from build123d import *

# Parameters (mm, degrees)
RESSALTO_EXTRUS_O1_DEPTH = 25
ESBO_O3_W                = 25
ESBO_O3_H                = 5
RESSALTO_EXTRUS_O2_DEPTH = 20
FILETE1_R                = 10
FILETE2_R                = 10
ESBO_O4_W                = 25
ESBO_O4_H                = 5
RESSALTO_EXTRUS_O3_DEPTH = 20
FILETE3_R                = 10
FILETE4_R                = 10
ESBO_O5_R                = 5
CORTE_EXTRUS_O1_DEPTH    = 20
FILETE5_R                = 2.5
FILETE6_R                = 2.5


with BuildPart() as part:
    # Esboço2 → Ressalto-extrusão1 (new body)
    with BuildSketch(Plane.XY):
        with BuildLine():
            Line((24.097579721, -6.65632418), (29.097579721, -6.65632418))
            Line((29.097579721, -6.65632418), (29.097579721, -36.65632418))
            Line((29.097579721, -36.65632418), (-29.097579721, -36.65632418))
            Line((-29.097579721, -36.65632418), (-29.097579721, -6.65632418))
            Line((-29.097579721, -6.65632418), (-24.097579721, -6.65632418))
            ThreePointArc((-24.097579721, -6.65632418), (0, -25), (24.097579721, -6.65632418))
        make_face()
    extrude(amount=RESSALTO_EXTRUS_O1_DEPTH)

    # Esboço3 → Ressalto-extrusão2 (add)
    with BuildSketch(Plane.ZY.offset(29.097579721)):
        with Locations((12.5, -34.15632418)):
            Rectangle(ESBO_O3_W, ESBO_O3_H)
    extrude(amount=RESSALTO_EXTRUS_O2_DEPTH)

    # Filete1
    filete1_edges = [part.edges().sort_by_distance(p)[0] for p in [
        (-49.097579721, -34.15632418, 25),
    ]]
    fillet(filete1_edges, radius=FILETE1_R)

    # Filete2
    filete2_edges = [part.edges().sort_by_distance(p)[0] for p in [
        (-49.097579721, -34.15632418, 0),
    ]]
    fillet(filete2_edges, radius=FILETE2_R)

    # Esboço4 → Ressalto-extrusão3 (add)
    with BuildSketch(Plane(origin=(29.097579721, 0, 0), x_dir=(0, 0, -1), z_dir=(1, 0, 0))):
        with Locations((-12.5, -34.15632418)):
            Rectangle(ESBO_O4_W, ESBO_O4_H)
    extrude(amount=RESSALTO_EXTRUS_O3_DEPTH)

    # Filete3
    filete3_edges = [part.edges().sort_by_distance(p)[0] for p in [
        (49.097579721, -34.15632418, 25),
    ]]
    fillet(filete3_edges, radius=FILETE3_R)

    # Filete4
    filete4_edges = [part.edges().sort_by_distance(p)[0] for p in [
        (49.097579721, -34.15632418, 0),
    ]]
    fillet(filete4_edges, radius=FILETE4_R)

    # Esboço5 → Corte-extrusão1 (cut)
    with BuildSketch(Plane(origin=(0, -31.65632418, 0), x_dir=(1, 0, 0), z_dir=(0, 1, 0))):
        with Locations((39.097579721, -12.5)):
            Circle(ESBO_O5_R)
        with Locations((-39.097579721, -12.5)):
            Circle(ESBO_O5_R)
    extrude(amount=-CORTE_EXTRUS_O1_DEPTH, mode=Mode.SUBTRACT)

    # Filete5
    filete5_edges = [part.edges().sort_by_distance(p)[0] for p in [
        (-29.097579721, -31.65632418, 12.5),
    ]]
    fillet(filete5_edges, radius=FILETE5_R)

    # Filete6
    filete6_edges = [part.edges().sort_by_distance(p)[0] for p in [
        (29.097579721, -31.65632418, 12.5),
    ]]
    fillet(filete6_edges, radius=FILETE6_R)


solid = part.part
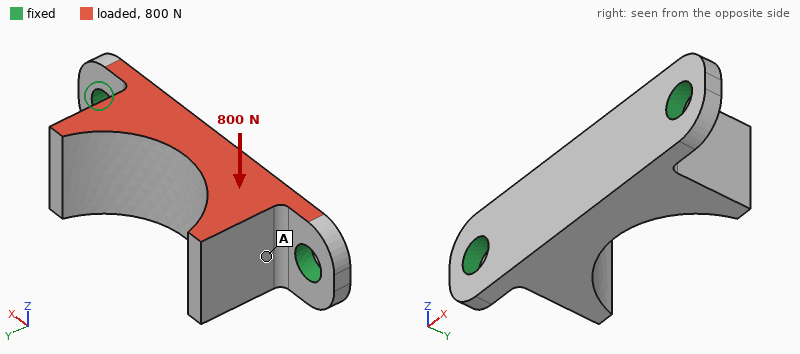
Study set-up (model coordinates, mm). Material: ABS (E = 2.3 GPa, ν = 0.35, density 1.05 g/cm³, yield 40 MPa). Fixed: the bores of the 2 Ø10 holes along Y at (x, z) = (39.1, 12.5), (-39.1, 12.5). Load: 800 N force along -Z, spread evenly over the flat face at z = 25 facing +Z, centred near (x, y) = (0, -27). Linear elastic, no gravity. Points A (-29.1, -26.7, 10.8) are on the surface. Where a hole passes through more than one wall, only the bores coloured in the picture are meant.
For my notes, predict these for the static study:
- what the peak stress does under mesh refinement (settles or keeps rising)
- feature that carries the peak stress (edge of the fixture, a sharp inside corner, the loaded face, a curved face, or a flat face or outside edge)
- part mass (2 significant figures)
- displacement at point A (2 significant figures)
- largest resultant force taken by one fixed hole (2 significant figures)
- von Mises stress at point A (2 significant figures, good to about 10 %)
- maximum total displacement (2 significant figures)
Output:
keeps rising
edge of the fixture
33 g
0.17 mm
400 N
4.4 MPa
0.55 mm
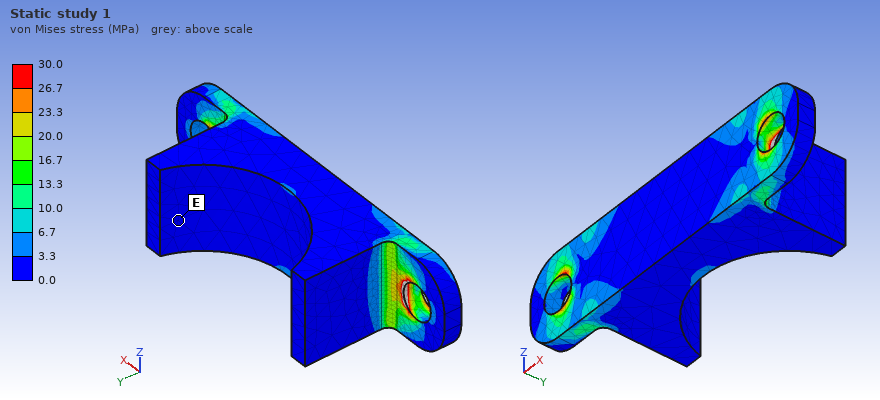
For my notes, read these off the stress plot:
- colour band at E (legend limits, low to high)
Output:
0.0 to 3.3 MPa
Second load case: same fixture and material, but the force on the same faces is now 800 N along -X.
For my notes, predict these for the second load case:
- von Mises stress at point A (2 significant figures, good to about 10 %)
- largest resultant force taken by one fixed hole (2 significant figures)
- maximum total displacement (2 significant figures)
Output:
1.4 MPa
430 N
94 µm
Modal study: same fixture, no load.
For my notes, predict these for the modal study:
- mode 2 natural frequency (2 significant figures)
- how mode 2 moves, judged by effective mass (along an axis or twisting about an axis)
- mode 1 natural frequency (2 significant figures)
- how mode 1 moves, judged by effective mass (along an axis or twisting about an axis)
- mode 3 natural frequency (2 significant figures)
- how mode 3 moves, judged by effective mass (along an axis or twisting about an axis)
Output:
1900 Hz
along Y
1300 Hz
along Z
3000 Hz
twisting about Y
